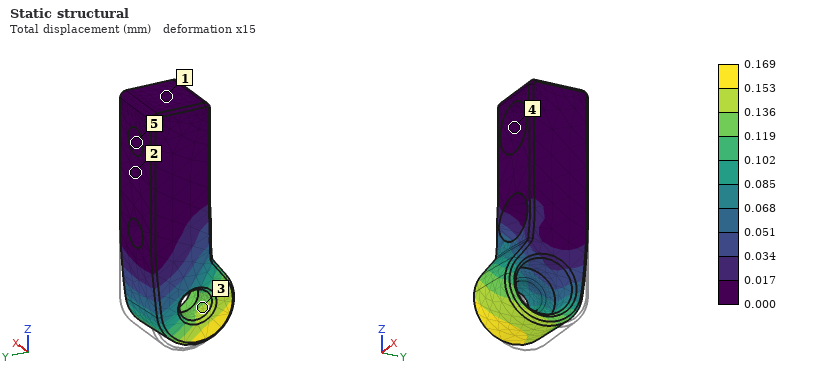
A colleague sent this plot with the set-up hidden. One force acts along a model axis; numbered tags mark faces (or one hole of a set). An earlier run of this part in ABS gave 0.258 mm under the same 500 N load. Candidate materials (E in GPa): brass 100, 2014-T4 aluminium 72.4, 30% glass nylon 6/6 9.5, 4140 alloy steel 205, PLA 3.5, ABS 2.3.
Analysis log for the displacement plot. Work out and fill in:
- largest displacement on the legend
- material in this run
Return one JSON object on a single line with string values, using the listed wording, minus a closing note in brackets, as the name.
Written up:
{"largest displacement on the legend": "0.169 mm", "material in this run": "PLA"}
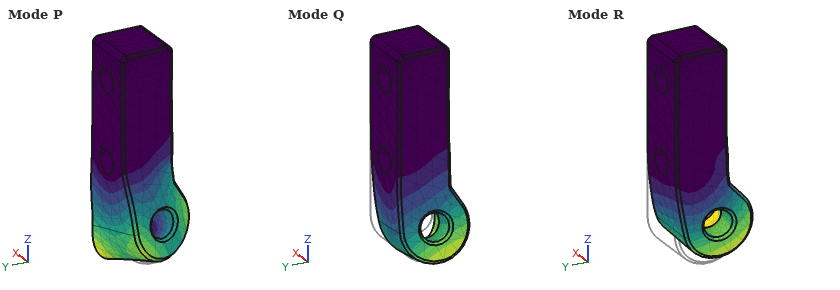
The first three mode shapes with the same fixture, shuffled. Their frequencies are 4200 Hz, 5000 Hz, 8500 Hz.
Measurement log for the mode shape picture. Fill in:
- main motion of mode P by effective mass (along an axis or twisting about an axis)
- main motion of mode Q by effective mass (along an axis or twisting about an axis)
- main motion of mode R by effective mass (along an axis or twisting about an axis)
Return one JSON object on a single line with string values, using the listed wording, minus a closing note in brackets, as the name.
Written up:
{"main motion of mode P by effective mass": "twisting about Z", "main motion of mode Q by effective mass": "along X", "main motion of mode R by effective mass": "along Y"}
